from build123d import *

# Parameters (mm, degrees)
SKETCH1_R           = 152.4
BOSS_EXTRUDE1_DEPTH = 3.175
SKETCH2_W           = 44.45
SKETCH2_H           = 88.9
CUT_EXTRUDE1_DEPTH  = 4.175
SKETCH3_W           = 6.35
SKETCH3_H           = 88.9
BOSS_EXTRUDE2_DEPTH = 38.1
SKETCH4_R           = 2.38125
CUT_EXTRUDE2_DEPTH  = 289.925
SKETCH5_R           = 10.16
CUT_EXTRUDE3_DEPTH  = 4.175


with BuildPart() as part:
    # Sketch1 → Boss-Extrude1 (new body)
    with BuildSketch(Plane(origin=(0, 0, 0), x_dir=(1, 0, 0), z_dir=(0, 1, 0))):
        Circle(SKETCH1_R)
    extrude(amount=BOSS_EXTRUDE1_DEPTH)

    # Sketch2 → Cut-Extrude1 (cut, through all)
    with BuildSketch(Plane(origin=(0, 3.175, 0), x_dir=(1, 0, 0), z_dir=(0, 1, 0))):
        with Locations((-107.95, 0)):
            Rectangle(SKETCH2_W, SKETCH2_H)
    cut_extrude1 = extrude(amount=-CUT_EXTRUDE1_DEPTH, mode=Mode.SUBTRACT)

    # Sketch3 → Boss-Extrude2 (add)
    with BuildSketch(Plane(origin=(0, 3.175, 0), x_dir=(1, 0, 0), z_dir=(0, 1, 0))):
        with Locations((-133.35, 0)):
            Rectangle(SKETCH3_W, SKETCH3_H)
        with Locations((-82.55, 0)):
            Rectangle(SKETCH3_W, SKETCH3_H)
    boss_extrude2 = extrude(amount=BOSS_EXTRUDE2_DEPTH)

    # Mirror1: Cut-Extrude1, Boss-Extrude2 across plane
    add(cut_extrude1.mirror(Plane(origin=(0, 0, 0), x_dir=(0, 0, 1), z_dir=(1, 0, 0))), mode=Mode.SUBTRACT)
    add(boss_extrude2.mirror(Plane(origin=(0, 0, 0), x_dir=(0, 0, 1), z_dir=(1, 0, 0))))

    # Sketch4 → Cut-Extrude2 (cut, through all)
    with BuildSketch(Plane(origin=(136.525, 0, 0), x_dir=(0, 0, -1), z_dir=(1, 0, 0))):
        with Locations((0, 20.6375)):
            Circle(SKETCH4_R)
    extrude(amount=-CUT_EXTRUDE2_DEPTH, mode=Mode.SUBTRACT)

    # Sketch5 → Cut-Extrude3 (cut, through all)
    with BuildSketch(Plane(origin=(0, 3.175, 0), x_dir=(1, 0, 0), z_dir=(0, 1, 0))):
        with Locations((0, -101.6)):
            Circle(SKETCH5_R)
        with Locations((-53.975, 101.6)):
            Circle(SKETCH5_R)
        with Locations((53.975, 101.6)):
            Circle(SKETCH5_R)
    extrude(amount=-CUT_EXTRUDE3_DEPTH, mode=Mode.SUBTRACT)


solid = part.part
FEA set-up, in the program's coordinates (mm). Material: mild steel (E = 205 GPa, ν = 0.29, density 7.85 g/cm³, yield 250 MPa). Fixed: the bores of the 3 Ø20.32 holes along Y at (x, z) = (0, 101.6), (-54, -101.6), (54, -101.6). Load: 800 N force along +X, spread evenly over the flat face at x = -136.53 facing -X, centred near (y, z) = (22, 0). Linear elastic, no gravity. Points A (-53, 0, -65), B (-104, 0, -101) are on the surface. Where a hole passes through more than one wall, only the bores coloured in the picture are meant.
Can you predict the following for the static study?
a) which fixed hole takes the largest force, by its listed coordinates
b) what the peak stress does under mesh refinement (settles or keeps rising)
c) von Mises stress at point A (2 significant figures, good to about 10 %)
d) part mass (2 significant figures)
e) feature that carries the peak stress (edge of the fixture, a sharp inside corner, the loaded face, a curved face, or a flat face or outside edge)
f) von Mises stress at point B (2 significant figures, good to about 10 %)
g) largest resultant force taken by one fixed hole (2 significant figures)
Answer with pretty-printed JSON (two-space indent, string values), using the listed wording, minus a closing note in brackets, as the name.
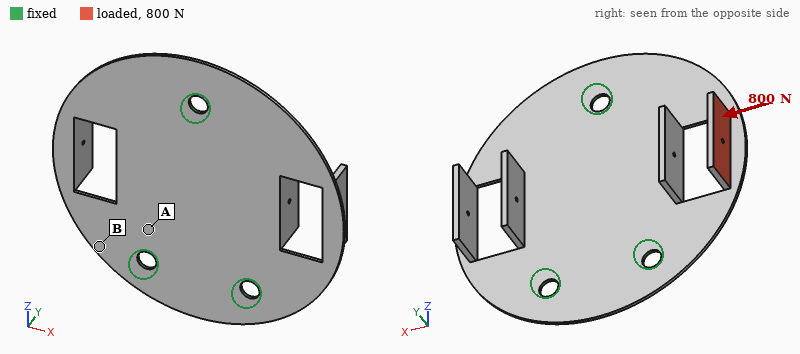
{
  "which fixed hole takes the largest force, by its listed coordinates": "(0, 101.6)",
  "what the peak stress does under mesh refinement": "keeps rising",
  "von Mises stress at point A": "26 MPa",
  "part mass": "2.3 kg",
  "feature that carries the peak stress": "a sharp inside corner",
  "von Mises stress at point B": "68 MPa",
  "largest resultant force taken by one fixed hole": "440 N"
}
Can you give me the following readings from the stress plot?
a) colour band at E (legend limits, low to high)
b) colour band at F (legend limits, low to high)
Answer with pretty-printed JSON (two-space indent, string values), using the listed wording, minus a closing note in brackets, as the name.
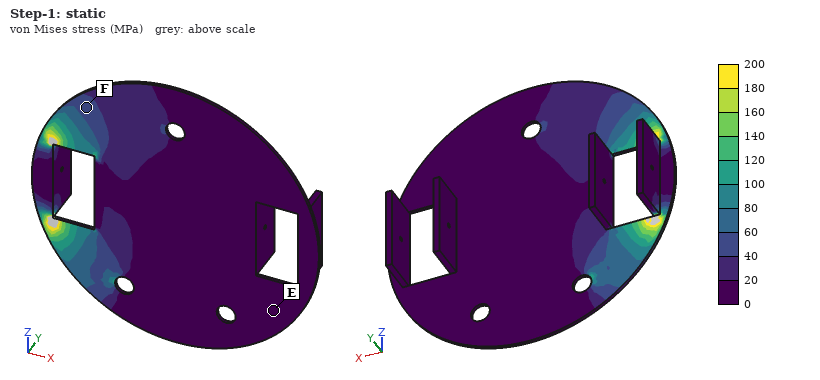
{
  "colour band at E": "0 to 20 MPa",
  "colour band at F": "40 to 60 MPa"
}
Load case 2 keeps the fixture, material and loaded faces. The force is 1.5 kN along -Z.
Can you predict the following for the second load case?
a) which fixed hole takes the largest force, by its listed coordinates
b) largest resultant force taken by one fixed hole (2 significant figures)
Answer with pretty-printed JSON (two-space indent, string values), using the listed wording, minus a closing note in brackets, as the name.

{
  "which fixed hole takes the largest force, by its listed coordinates": "(-54, -101.6)",
  "largest resultant force taken by one fixed hole": "1.2 kN"
}
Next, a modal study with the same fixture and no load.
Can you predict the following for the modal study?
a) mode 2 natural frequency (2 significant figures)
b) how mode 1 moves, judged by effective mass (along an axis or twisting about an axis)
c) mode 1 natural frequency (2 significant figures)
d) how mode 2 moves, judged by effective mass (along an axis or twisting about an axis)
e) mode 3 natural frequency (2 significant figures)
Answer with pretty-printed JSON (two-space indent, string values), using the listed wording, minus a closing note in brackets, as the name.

{
  "mode 2 natural frequency": "140 Hz",
  "how mode 1 moves, judged by effective mass": "twisting about Z",
  "mode 1 natural frequency": "140 Hz",
  "how mode 2 moves, judged by effective mass": "along Y",
  "mode 3 natural frequency": "350 Hz"
}
